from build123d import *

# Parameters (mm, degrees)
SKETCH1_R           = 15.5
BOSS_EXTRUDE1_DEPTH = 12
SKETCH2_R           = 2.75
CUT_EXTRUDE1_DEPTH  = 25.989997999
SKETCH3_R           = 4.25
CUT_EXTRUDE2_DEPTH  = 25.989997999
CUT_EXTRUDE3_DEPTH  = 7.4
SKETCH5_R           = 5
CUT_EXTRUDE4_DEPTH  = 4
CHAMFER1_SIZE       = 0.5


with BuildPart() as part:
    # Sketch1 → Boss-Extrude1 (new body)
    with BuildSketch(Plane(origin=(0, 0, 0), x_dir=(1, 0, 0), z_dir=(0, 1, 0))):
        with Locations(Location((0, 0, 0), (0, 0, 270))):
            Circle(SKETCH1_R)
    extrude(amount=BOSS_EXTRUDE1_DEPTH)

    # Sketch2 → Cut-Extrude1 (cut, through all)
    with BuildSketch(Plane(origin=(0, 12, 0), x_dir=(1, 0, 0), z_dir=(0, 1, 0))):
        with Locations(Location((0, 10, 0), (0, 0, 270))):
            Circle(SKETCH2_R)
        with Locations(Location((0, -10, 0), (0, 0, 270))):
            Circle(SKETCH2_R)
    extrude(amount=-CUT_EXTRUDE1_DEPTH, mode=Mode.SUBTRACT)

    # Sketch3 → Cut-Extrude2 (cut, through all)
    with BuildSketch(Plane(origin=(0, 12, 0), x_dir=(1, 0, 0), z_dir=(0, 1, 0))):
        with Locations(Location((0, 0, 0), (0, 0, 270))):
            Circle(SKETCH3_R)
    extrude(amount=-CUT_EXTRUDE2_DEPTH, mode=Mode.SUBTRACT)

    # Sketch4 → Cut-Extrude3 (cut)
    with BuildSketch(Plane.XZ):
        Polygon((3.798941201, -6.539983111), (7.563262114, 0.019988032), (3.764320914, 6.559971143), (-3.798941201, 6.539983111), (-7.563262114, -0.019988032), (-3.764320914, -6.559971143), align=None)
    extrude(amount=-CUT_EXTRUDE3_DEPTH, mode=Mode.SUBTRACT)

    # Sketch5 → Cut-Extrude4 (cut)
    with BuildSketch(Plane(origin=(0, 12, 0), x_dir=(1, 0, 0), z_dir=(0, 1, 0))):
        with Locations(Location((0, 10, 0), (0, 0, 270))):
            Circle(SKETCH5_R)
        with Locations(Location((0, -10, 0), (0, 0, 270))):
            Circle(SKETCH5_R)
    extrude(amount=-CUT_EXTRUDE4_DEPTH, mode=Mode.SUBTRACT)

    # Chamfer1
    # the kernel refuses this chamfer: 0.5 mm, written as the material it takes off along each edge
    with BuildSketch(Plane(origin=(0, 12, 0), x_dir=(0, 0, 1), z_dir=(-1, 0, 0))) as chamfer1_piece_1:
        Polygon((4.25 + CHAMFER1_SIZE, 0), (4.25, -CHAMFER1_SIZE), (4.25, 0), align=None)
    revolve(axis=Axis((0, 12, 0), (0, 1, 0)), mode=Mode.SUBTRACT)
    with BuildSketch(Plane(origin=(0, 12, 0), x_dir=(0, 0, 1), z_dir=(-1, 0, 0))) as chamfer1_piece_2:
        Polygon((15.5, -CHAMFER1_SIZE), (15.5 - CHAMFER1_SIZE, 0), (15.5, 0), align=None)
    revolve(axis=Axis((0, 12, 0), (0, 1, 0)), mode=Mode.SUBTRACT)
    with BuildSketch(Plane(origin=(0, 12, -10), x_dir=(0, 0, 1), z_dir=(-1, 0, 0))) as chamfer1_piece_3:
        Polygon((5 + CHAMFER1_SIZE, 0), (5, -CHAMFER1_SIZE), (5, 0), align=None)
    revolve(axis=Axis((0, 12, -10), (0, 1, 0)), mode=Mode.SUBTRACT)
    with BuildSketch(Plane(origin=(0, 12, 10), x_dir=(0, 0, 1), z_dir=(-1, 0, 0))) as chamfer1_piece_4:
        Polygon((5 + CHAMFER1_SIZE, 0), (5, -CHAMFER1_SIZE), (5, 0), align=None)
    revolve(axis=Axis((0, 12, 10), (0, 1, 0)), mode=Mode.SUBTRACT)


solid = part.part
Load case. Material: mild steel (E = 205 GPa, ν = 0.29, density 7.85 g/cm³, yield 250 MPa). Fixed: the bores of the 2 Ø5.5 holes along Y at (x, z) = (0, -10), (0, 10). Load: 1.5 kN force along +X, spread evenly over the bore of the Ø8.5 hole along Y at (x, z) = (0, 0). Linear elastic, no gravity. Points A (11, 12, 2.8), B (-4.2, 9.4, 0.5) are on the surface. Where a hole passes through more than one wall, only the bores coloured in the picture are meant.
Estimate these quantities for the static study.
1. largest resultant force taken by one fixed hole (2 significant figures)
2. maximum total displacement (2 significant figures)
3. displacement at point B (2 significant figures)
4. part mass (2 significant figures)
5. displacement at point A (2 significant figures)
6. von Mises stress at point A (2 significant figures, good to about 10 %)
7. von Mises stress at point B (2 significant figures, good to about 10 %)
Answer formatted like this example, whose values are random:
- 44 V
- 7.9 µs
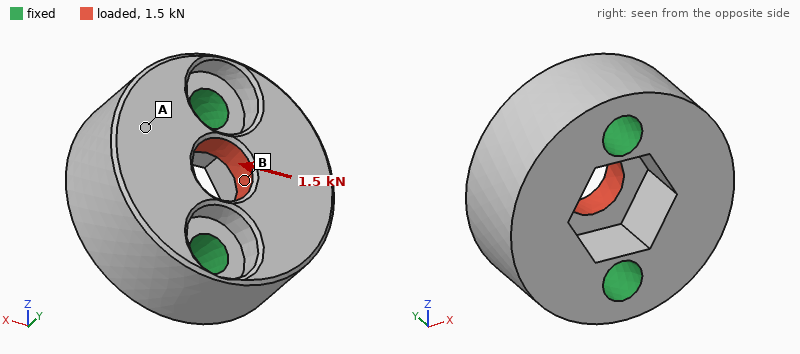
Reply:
- 750 N
- 2.1 µm
- 1.4 µm
- 52 g
- 1.7 µm
- 5.5 MPa
- 10 MPa
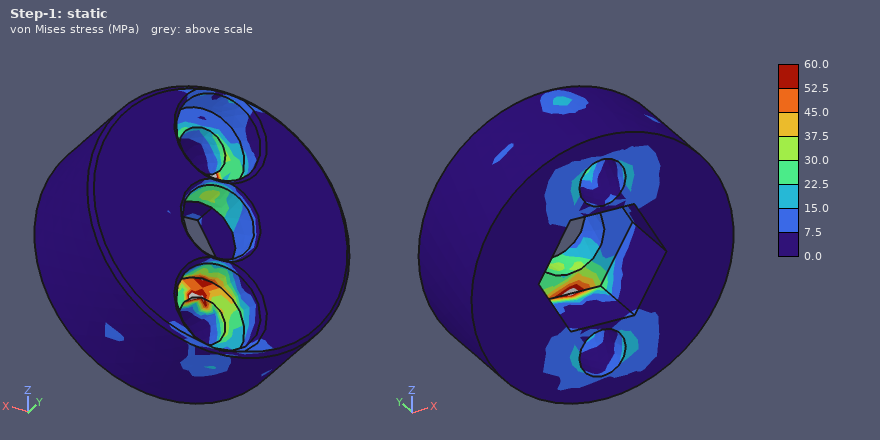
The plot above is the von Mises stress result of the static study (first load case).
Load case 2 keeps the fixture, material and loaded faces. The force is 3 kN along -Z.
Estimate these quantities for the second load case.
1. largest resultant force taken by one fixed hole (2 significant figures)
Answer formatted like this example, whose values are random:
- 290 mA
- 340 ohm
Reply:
- 1.6 kN
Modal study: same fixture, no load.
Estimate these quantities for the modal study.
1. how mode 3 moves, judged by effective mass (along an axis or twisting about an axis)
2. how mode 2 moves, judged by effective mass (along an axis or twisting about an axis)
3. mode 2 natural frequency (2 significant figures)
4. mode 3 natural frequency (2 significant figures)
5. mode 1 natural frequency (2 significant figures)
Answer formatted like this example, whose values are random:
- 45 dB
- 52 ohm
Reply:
- twisting about Y
- along Y
- 26 kHz
- 41 kHz
- 22 kHz
